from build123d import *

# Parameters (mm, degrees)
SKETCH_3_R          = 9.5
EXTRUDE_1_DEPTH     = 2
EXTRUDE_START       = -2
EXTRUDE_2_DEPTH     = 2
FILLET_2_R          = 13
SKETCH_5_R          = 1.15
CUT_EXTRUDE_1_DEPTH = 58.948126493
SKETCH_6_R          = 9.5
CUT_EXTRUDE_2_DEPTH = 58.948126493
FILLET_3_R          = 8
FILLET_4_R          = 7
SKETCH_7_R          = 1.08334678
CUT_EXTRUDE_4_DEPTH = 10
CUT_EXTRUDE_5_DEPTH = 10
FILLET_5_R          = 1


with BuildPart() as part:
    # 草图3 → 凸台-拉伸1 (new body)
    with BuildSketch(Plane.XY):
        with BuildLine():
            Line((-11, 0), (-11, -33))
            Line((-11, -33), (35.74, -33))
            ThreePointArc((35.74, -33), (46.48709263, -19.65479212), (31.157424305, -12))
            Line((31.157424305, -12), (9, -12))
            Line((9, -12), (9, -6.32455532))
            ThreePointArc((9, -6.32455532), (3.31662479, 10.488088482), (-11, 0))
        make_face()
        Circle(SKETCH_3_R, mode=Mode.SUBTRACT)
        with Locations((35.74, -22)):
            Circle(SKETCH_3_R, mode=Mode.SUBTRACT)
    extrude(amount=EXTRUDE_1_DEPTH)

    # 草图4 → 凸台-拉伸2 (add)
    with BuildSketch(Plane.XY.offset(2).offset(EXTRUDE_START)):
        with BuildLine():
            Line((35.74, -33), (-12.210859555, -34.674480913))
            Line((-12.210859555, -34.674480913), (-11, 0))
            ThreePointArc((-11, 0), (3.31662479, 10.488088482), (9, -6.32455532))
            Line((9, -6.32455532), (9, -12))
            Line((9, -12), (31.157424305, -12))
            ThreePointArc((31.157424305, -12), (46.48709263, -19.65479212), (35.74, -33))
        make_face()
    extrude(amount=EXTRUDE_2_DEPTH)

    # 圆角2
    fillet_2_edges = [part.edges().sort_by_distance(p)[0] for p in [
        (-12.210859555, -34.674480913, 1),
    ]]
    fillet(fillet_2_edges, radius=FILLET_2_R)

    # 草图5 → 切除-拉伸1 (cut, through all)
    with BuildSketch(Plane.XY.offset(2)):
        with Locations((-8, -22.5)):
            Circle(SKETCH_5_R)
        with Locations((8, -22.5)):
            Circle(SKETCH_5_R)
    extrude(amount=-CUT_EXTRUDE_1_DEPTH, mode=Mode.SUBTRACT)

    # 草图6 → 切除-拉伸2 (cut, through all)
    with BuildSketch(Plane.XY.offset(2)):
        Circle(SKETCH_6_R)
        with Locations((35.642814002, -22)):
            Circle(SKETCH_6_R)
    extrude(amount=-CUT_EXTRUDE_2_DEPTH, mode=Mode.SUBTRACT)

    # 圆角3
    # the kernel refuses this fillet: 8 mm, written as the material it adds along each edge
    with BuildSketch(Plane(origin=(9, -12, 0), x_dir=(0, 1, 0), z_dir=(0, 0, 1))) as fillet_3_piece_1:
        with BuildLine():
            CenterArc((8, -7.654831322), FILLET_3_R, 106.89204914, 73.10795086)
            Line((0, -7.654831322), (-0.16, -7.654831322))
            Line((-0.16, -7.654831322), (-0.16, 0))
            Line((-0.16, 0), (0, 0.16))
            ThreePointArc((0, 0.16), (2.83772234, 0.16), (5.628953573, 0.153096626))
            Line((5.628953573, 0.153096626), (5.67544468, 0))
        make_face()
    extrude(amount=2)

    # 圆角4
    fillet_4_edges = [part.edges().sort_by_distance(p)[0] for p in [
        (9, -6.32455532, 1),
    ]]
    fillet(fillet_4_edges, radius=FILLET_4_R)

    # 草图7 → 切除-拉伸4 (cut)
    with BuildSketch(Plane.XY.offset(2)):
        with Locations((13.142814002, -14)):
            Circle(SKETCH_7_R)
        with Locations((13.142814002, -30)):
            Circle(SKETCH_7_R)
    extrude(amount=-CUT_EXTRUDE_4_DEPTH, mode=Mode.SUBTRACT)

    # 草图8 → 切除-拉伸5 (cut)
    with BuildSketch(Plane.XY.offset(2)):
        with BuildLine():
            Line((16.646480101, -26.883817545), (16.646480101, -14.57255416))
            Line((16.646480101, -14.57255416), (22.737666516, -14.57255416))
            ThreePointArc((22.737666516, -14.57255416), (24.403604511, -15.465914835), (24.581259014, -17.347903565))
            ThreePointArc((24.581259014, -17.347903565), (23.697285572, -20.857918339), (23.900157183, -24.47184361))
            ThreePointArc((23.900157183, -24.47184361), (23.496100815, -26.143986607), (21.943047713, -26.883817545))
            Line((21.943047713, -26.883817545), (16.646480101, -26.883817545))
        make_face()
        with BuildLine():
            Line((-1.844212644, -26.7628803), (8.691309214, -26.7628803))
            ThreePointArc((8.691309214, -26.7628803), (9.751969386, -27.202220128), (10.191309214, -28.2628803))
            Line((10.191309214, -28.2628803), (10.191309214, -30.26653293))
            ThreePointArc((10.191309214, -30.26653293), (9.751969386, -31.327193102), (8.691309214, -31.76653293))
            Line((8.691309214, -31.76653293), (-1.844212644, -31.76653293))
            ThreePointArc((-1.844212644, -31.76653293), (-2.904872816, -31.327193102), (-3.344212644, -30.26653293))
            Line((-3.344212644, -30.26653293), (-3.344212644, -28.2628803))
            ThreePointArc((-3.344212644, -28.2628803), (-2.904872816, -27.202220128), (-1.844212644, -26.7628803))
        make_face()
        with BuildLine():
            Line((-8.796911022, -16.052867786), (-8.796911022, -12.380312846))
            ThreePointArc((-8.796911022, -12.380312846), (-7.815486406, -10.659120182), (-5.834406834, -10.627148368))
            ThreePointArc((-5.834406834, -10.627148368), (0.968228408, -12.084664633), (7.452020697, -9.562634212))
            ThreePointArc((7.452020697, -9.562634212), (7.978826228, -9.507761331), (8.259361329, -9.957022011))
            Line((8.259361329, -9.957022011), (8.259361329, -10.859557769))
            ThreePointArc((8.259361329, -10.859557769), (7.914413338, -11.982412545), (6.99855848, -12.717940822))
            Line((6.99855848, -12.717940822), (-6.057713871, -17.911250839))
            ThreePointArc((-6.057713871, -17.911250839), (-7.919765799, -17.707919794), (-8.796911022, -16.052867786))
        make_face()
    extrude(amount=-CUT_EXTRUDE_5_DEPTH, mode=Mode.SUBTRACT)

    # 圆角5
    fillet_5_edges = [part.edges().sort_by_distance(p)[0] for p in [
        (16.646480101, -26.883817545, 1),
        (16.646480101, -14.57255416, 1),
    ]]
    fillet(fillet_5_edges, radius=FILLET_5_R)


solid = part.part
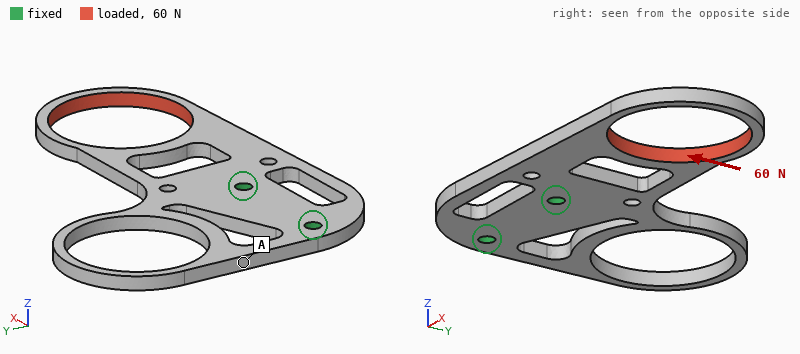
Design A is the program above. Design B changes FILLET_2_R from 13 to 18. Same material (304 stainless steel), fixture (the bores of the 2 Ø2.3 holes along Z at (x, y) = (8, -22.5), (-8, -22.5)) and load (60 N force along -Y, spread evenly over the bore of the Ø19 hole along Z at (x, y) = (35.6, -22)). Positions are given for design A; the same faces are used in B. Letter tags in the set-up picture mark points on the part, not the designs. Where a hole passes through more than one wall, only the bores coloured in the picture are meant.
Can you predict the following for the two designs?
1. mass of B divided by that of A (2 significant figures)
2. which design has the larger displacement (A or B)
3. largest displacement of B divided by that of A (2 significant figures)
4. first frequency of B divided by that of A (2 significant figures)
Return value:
0.95
B
1.1
1.00
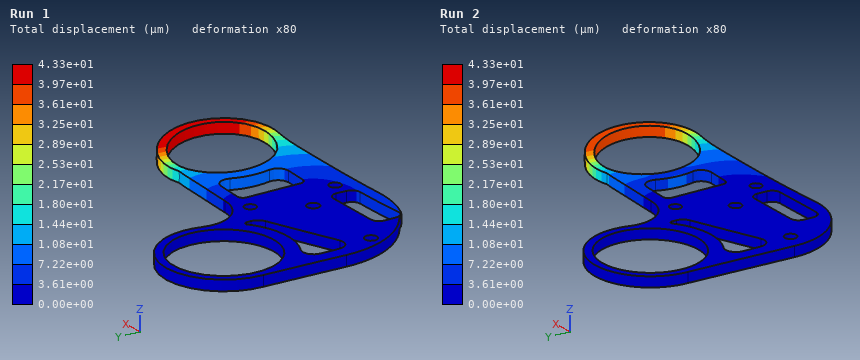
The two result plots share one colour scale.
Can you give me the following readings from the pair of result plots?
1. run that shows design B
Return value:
Run 1
